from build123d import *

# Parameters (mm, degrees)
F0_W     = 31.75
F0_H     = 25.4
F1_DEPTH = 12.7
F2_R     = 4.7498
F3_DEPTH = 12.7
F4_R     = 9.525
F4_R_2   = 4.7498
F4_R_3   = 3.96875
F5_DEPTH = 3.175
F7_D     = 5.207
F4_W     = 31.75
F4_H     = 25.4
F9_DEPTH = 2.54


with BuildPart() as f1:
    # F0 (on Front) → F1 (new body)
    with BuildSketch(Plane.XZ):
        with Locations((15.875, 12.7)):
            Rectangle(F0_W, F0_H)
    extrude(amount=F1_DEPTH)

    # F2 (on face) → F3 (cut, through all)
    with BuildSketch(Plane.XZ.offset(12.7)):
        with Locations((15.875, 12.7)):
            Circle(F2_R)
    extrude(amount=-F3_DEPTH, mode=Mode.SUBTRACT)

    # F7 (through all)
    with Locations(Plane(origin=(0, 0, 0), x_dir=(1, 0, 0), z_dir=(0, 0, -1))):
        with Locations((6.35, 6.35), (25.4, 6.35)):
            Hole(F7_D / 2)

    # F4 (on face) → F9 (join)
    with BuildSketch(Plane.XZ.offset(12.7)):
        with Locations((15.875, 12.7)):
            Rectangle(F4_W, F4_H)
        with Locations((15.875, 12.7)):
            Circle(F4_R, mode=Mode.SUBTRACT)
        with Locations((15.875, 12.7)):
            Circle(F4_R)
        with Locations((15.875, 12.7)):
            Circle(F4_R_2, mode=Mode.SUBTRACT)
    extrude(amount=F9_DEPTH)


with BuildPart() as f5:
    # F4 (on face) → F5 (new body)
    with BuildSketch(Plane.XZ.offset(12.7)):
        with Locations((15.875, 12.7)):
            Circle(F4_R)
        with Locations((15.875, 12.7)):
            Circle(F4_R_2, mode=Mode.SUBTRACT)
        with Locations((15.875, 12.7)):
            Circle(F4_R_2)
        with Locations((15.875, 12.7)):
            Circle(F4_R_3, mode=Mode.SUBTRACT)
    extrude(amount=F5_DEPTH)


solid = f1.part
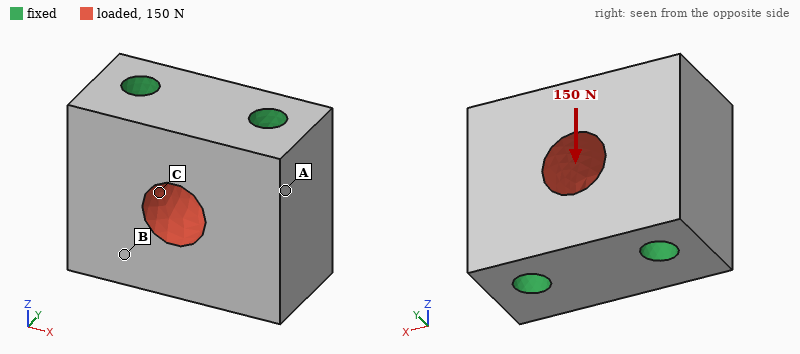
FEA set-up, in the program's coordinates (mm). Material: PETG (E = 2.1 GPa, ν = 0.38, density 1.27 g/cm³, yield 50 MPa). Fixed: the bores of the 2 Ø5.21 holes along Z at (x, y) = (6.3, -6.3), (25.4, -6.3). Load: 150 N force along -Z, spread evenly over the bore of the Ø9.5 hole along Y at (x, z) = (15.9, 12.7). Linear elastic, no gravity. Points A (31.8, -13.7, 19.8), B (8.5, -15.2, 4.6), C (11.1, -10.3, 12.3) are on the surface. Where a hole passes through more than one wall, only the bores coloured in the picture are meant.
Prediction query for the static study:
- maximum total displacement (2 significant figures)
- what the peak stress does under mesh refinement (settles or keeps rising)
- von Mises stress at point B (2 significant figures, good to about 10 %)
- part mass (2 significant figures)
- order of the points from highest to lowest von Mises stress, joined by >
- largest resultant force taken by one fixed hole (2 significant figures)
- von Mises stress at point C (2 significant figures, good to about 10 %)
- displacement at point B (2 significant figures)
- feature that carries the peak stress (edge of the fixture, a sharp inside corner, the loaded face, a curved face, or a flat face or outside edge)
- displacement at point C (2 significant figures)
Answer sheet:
2.8 µm
keeps rising
0.22 MPa
13 g
C > B > A
75 N
0.63 MPa
1.1 µm
edge of the fixture
1.6 µm
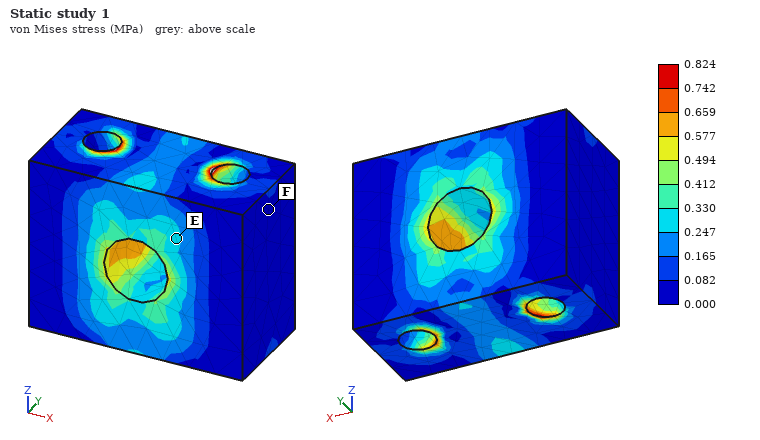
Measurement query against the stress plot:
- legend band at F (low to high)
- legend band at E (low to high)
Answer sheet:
0.000 to 0.082 MPa
0.247 to 0.330 MPa
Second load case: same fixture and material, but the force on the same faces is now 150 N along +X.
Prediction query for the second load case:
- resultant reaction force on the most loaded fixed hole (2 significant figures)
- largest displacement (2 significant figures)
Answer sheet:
75 N
2.1 µm
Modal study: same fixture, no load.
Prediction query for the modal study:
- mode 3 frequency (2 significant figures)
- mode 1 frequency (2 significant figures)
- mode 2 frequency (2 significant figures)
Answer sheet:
19 kHz
18 kHz
19 kHz
